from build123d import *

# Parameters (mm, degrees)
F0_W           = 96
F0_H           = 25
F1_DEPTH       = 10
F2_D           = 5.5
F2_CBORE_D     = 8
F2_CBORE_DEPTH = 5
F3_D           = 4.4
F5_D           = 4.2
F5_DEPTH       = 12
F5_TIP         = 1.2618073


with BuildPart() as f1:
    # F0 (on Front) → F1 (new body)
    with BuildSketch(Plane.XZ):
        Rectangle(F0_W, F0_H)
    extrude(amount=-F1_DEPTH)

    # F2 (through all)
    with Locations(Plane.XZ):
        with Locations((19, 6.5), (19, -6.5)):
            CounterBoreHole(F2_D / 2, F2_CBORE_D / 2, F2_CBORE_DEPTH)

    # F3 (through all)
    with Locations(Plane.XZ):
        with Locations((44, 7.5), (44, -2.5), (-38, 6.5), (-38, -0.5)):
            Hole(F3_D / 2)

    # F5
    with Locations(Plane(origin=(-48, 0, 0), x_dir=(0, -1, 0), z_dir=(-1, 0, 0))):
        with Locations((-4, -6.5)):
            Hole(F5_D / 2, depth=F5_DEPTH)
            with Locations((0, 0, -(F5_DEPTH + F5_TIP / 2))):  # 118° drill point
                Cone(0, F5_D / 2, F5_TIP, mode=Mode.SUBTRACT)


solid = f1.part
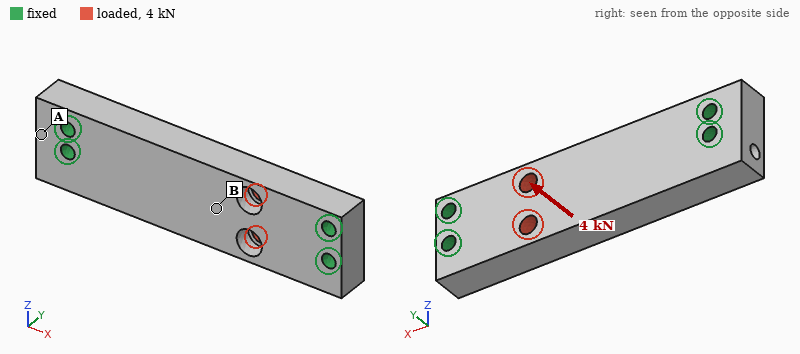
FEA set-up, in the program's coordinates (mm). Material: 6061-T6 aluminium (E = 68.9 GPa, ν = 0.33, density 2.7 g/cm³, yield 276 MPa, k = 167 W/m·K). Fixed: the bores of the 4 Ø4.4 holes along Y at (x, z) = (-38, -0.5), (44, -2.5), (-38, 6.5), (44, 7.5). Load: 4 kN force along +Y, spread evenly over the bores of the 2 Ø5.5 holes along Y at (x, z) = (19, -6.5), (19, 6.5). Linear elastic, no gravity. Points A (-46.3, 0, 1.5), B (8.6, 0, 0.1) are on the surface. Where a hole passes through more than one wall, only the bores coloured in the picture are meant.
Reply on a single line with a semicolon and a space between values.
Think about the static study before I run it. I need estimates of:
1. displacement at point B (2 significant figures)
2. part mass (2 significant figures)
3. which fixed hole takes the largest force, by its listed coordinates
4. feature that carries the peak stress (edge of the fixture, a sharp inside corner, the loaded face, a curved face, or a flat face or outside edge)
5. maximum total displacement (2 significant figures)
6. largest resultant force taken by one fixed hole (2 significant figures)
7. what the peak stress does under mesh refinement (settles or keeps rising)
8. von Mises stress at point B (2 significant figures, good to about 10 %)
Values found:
70 µm; 61 g; (44, -2.5); edge of the fixture; 79 µm; 1.9 kN; keeps rising; 45 MPa
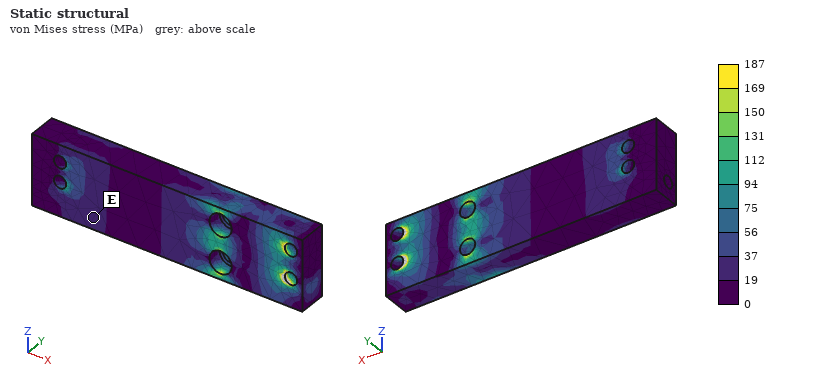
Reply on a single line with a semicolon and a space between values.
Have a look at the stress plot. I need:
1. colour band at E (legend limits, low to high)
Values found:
19 to 37 MPa
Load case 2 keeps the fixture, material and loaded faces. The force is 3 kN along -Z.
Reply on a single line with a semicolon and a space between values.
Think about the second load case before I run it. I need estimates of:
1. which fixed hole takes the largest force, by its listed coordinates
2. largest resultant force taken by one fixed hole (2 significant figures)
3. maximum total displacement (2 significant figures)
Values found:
(44, 7.5); 2.5 kN; 26 µm
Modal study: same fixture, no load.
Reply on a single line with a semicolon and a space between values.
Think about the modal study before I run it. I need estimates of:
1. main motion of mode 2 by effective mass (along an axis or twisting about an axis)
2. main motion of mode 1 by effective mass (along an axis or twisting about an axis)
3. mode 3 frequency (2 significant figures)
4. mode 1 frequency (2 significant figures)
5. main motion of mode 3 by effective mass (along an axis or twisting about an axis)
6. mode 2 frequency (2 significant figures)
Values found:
along Z; along Y; 13 kHz; 7100 Hz; twisting about X; 11 kHz
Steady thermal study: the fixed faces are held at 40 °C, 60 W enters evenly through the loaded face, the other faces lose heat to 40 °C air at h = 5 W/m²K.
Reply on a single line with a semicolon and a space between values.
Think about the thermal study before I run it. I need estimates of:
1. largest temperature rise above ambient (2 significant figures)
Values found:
29 K
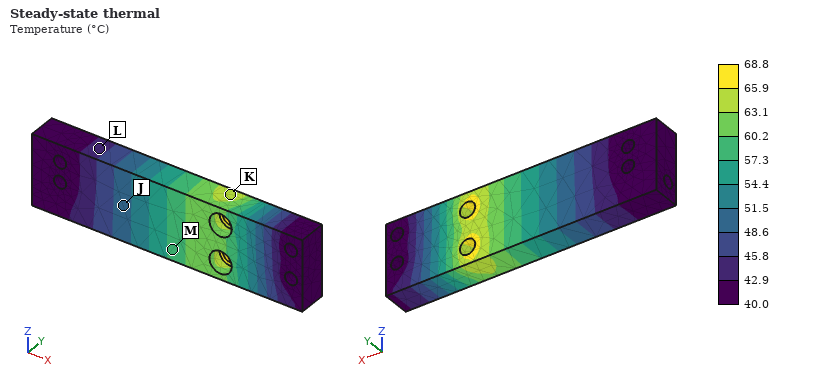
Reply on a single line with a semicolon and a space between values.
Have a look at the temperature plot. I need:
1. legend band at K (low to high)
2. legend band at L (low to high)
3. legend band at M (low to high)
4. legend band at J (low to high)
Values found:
63.1 to 65.9 °C; 42.9 to 45.8 °C; 57.3 to 60.2 °C; 48.6 to 51.5 °C
